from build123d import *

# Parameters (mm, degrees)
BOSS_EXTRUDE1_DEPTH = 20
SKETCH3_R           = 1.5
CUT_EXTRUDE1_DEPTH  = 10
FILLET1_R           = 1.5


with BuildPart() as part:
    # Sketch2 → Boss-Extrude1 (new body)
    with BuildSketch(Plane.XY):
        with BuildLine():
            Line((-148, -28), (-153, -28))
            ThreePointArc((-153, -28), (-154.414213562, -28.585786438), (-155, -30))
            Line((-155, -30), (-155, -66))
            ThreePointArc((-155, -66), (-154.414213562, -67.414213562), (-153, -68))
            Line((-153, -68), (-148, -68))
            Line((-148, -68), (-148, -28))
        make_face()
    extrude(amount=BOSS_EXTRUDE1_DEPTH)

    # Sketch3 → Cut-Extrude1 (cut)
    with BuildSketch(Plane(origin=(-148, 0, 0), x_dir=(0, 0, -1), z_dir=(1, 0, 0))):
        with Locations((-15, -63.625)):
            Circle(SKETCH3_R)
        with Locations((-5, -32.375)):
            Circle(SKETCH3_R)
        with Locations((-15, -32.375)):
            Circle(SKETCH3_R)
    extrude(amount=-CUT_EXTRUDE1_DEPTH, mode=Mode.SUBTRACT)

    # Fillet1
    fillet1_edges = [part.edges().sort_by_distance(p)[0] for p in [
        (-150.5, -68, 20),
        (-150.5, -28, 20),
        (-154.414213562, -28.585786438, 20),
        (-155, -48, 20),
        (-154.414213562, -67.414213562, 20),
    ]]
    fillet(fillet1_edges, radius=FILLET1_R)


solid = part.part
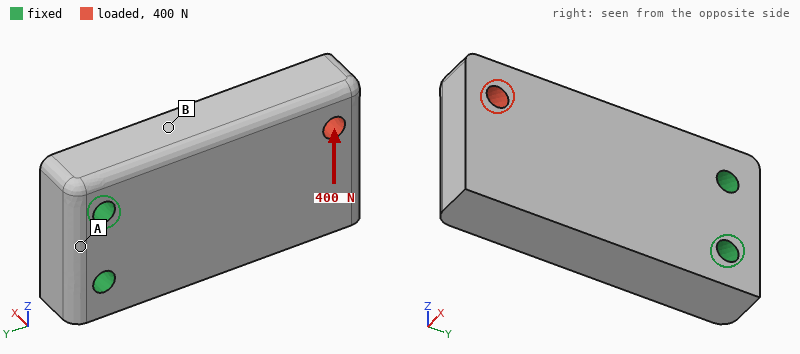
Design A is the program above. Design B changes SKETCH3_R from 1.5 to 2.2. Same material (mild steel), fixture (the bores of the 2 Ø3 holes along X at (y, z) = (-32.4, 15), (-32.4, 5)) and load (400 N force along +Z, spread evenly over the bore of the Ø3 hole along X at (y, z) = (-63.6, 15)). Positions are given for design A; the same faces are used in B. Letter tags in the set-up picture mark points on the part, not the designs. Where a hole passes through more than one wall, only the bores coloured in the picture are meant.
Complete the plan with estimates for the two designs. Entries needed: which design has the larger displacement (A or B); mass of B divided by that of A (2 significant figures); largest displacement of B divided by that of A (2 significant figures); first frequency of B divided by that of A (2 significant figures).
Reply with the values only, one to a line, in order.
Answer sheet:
A
0.97
0.89
1.1
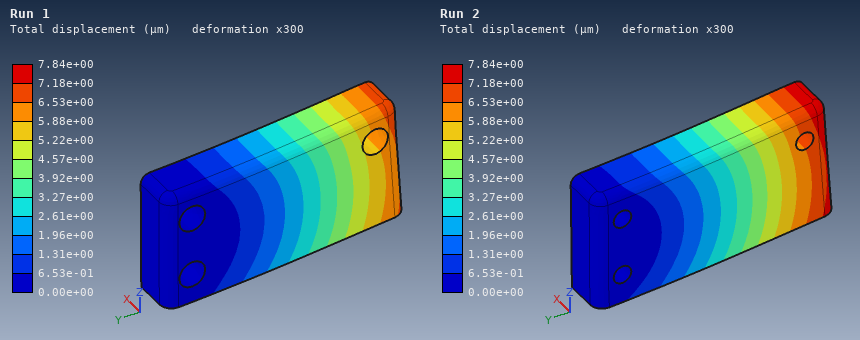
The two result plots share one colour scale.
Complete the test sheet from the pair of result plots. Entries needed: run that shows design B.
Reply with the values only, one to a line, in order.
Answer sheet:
Run 1
